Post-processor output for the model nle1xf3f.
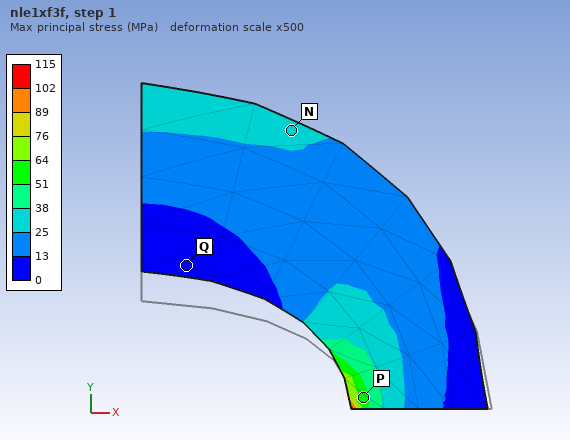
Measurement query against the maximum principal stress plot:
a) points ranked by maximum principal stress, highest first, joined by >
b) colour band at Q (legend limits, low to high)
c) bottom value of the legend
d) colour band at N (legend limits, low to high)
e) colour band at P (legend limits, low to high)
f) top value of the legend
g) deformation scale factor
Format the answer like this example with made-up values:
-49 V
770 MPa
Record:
P > N > Q
0 to 13 MPa
0 MPa
25 to 38 MPa
51 to 64 MPa
115 MPa
500
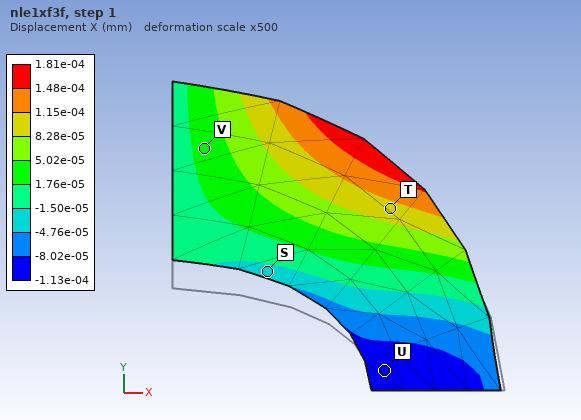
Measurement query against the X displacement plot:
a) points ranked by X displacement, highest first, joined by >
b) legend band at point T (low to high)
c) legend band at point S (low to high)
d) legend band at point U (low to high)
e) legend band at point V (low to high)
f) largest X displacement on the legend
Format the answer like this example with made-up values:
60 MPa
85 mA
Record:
T > V > S > U
8.28e-05 to 1.15e-04 mm
-4.76e-05 to -1.50e-05 mm
-1.13e-04 to -8.02e-05 mm
1.76e-05 to 5.02e-05 mm
1.81e-04 mm
